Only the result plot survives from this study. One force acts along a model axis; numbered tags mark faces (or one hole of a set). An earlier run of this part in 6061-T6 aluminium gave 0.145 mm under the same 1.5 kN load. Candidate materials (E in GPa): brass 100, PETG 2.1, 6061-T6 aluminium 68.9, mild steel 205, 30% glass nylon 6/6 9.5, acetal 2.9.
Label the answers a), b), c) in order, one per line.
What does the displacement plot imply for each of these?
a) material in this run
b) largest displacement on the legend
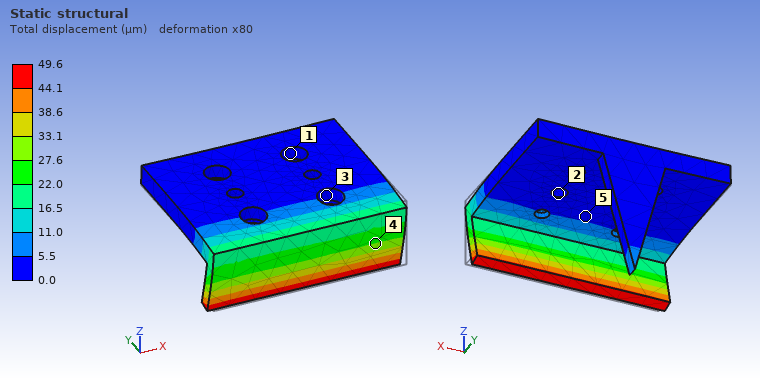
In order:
a) mild steel
b) 49.6 µm
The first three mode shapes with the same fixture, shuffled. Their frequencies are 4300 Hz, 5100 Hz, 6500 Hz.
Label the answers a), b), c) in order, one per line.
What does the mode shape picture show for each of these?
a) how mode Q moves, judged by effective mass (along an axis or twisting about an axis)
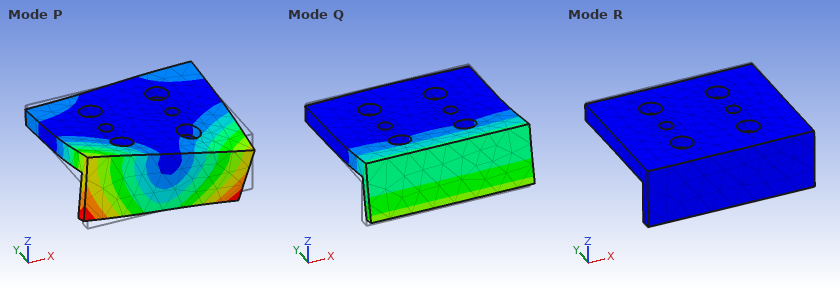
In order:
a) along Z
